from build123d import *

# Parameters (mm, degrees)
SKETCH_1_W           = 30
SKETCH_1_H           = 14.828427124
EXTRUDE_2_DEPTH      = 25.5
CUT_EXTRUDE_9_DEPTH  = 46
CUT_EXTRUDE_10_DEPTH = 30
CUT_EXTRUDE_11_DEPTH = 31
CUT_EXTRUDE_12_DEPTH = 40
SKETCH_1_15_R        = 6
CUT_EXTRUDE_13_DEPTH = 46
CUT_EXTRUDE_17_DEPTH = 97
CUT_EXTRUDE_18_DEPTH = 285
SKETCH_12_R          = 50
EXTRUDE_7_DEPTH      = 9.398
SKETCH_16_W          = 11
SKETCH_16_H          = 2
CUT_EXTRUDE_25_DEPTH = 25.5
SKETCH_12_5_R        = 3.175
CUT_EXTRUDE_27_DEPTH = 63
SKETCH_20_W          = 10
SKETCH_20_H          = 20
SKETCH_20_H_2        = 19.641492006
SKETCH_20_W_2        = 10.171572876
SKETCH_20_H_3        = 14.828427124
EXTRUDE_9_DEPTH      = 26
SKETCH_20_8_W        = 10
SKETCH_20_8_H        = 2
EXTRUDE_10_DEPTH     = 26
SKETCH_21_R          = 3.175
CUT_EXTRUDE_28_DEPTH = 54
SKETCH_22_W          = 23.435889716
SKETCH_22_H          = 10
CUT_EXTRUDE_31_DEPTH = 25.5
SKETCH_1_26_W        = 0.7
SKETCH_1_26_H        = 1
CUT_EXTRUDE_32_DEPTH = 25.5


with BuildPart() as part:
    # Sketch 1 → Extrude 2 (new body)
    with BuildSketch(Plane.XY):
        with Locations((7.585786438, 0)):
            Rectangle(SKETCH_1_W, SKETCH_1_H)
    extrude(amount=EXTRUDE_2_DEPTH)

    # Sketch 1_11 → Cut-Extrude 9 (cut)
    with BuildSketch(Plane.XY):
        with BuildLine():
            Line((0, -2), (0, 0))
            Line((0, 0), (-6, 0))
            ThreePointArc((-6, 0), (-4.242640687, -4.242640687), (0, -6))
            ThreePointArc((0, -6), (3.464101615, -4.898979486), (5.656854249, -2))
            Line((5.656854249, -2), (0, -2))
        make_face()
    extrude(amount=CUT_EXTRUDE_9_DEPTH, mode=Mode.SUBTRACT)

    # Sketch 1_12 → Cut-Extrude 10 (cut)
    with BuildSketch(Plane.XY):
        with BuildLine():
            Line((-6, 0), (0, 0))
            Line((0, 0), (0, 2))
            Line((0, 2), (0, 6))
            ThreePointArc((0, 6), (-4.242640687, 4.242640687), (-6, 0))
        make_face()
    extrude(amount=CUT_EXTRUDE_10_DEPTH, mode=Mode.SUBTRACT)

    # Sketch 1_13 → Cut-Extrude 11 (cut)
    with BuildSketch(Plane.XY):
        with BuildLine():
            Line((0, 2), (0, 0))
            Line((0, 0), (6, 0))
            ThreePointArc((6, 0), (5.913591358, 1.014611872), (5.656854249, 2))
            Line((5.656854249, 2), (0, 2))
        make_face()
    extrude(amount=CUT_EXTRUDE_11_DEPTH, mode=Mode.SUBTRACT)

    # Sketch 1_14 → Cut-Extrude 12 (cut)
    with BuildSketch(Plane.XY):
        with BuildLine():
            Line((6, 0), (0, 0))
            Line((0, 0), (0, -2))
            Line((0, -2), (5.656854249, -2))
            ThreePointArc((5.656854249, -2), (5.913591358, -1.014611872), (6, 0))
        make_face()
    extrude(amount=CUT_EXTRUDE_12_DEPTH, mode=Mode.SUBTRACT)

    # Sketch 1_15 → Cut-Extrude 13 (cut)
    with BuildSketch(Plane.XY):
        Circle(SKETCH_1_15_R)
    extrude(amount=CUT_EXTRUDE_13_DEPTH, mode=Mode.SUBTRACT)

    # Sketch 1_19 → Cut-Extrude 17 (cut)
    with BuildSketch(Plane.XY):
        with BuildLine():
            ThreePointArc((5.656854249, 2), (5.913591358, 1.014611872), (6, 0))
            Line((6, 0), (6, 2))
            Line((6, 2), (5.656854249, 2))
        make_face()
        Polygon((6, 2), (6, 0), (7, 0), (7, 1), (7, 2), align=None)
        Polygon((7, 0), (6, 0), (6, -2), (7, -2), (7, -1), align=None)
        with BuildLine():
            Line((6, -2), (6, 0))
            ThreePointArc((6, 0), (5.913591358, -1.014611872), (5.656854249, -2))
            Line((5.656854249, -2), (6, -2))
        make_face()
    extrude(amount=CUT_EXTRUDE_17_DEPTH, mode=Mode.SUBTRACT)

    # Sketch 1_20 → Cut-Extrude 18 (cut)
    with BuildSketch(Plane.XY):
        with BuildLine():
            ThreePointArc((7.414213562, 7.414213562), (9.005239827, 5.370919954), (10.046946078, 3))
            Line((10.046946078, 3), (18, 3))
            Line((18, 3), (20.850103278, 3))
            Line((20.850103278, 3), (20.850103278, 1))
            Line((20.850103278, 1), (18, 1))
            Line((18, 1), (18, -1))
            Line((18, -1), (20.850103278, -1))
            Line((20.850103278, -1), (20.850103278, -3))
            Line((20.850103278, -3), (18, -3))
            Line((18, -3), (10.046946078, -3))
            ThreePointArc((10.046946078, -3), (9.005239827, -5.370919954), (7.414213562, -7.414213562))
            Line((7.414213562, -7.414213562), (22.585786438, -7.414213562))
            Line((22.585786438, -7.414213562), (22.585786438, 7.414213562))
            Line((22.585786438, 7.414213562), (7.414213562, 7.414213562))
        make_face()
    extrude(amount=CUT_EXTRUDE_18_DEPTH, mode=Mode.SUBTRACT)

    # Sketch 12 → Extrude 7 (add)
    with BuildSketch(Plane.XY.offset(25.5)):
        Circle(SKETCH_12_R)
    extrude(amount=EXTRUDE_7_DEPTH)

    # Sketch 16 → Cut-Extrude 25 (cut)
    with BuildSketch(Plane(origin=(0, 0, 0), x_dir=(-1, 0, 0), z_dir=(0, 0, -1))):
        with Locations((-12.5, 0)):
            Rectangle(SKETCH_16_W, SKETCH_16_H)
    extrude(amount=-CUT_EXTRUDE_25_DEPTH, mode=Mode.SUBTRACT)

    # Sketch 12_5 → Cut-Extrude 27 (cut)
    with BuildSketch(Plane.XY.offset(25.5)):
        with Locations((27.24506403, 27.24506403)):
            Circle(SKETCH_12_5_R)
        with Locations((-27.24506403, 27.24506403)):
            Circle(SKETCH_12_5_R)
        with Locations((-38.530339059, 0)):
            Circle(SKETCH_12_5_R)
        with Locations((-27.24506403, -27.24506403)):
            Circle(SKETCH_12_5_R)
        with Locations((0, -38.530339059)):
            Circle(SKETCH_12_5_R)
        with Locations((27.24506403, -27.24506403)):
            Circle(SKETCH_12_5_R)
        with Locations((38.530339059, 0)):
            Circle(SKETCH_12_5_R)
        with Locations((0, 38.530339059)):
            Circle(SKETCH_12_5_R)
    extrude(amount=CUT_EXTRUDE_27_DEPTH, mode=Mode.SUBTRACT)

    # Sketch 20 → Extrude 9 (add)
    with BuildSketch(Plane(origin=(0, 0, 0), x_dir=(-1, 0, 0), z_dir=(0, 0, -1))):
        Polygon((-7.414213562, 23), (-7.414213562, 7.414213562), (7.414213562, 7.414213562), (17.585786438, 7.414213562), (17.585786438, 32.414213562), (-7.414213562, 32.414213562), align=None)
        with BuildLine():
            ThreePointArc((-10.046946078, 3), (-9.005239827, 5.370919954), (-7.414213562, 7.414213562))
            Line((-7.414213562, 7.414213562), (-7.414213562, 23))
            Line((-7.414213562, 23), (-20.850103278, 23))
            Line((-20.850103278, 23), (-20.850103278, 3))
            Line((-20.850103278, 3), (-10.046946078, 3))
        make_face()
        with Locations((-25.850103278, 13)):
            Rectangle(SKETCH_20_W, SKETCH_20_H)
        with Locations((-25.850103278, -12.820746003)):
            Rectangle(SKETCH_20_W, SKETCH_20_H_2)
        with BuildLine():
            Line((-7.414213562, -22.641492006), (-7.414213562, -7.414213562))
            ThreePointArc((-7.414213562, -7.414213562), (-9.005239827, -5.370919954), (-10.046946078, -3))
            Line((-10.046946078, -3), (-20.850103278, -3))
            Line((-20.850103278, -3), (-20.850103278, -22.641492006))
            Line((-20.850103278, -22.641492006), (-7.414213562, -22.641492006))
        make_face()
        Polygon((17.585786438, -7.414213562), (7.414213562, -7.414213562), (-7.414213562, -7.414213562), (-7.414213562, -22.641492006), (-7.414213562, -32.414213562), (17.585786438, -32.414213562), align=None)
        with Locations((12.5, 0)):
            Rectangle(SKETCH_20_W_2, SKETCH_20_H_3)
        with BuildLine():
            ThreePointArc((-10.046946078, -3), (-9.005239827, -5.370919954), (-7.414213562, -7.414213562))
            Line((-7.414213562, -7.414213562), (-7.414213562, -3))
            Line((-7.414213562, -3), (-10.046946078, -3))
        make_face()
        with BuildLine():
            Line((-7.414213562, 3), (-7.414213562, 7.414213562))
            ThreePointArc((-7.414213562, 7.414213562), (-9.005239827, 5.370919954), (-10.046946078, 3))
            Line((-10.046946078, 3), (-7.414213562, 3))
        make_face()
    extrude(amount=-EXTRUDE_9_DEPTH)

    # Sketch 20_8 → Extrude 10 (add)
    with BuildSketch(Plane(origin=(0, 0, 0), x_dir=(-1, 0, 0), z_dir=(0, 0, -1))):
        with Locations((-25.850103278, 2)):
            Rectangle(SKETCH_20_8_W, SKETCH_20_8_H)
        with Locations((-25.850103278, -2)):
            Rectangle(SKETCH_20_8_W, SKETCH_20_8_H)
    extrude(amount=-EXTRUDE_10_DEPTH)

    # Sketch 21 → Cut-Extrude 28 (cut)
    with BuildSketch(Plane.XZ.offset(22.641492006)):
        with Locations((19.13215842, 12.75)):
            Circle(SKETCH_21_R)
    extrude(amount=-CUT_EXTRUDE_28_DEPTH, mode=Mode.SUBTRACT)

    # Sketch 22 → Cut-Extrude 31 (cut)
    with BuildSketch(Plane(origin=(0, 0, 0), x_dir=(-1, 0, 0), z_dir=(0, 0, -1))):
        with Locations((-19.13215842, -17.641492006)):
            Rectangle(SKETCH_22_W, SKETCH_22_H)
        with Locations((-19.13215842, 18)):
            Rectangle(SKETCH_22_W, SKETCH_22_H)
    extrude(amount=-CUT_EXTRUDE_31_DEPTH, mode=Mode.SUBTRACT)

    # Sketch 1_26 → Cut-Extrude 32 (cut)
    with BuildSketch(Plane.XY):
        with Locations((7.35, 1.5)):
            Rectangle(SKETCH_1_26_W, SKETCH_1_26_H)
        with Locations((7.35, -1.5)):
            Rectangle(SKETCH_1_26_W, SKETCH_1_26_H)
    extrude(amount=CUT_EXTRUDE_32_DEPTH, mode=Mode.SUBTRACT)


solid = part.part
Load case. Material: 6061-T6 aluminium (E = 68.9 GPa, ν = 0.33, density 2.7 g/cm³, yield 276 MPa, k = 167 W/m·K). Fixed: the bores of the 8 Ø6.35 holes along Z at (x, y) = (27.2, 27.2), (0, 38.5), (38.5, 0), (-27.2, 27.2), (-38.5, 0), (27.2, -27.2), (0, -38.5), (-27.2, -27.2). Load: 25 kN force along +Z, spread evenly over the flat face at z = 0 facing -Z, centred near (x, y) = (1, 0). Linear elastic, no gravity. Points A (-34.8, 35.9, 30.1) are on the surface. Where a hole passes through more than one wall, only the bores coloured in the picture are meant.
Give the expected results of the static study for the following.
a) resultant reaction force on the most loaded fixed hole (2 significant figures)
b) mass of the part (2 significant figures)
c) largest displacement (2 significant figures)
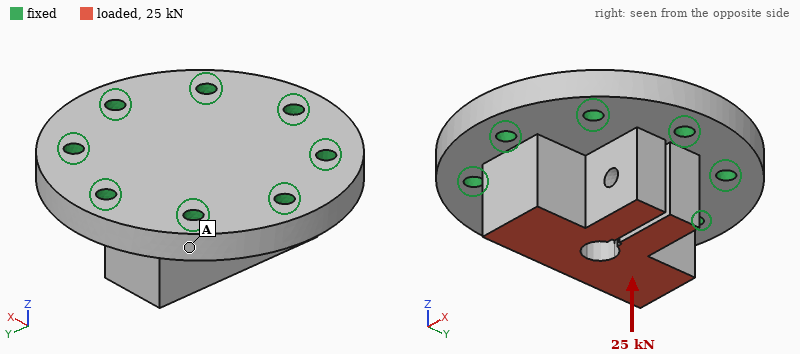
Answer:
4.9 kN
330 g
29 µm
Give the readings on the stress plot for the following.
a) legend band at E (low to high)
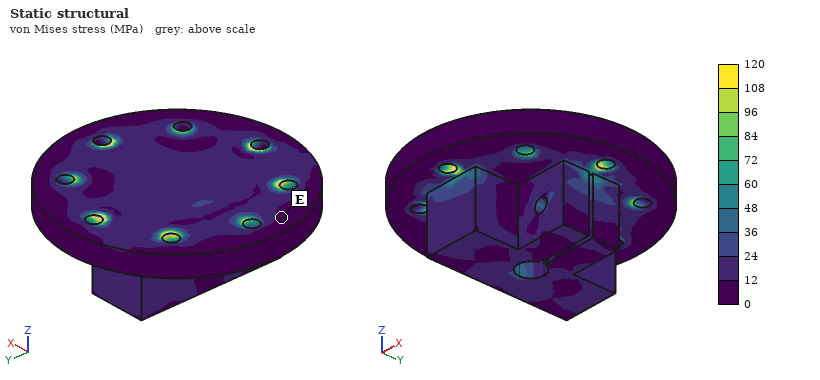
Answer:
0 to 12 MPa
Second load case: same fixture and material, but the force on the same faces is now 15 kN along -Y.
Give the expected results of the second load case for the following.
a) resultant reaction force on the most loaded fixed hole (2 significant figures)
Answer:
5.5 kN
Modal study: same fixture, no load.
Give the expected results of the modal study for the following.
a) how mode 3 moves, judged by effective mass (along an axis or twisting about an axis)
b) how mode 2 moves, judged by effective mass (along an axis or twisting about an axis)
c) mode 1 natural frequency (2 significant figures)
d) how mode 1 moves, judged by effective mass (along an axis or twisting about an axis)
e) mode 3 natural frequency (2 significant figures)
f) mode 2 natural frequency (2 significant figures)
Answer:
along Y
along X
11 kHz
along Z
14 kHz
13 kHz
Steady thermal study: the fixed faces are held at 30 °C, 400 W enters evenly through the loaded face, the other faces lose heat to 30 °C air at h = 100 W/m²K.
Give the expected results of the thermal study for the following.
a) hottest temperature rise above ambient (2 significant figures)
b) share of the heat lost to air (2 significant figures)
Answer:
51 K
9.7 %
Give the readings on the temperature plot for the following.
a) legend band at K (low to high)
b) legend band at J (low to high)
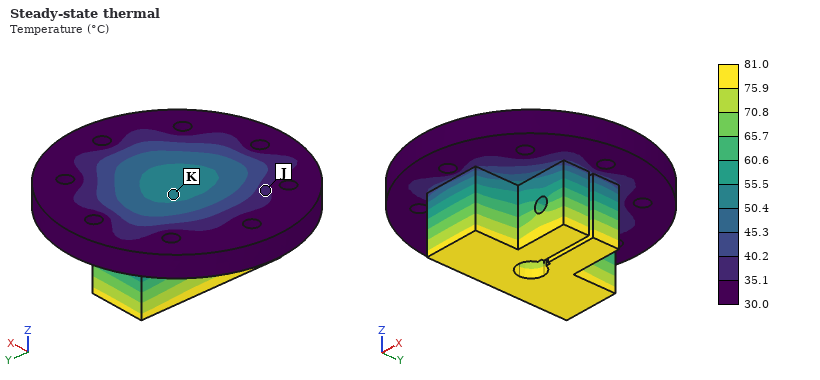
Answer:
50.4 to 55.5 °C
35.1 to 40.2 °C
